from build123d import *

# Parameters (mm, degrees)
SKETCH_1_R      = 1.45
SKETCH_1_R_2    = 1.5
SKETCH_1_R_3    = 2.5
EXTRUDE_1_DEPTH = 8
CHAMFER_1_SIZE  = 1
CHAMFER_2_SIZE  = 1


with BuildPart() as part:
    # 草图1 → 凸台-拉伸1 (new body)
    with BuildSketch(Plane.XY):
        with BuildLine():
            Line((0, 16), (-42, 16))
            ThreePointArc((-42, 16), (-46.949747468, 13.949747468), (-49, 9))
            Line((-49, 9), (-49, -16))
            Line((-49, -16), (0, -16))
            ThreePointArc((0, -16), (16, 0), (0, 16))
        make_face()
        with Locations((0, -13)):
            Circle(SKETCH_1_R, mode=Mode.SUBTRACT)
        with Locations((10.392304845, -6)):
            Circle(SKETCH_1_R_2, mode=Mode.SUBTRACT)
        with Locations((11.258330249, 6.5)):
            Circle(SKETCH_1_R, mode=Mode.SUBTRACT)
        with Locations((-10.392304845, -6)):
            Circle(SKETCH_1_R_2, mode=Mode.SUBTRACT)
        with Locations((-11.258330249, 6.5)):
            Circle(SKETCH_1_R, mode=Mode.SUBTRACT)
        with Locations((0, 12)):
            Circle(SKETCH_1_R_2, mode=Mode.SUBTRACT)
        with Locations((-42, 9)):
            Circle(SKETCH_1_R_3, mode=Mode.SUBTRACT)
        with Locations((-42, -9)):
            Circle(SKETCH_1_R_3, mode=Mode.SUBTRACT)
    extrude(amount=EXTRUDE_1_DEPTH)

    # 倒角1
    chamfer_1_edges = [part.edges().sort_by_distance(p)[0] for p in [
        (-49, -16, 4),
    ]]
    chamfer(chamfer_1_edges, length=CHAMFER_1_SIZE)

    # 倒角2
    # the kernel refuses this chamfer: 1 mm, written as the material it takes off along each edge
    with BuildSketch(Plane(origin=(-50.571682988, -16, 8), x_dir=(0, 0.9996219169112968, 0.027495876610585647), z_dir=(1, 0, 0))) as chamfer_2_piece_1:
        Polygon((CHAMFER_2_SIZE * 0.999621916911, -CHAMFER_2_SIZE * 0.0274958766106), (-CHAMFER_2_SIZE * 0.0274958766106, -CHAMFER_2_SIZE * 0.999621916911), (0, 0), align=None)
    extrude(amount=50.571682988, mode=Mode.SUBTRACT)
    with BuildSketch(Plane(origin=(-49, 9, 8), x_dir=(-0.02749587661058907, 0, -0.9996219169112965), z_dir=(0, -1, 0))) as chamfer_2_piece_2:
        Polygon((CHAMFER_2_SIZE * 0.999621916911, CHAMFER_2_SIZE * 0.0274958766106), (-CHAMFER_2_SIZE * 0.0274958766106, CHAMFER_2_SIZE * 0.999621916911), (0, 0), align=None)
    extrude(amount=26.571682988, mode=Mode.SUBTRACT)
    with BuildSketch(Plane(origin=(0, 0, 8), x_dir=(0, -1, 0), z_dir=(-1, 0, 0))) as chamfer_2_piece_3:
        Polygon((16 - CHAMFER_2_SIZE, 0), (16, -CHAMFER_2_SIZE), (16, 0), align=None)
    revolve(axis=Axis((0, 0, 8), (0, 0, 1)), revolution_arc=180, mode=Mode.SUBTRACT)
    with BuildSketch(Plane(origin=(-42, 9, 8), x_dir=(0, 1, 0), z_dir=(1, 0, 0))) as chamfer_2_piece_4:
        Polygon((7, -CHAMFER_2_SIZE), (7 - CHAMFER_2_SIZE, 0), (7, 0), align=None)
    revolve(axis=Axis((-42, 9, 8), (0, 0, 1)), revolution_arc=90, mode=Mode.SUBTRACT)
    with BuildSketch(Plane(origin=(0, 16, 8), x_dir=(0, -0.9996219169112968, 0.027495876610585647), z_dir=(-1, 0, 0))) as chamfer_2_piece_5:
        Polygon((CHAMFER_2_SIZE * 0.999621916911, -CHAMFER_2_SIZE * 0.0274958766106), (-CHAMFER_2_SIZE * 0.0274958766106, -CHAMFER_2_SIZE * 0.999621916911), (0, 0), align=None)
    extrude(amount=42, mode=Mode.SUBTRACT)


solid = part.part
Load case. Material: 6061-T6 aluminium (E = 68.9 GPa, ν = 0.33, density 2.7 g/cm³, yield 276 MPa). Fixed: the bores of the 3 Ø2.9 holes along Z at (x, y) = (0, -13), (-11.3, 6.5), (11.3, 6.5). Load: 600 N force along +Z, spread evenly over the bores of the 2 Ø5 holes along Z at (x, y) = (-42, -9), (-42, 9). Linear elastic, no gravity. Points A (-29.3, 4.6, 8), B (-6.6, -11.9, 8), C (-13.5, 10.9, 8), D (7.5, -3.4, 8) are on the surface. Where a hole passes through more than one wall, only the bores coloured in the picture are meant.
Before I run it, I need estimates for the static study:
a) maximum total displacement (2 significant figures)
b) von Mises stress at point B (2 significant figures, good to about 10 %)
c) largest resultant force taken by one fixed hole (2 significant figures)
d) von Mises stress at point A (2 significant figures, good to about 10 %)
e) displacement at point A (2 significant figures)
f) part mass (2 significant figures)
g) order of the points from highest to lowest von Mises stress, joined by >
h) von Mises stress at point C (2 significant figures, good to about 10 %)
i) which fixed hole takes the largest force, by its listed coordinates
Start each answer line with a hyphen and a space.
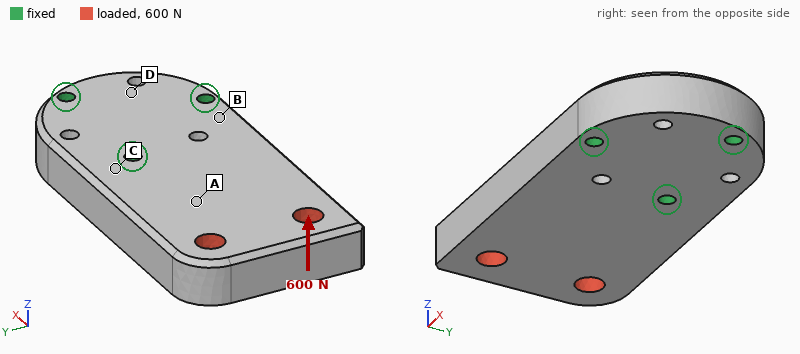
- 0.13 mm
- 33 MPa
- 910 N
- 22 MPa
- 0.043 mm
- 40 g
- C > B > A > D
- 44 MPa
- (-11.3, 6.5)
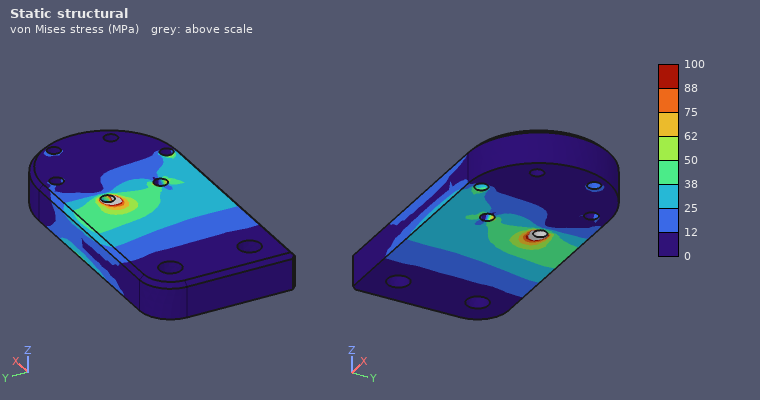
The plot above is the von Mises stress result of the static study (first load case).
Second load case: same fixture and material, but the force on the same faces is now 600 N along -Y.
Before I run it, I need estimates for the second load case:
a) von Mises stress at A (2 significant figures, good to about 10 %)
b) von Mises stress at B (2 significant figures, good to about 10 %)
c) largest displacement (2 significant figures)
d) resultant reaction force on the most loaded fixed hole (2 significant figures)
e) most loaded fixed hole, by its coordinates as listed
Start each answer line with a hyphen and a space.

- 5.8 MPa
- 12 MPa
- 15 µm
- 970 N
- (-11.3, 6.5)
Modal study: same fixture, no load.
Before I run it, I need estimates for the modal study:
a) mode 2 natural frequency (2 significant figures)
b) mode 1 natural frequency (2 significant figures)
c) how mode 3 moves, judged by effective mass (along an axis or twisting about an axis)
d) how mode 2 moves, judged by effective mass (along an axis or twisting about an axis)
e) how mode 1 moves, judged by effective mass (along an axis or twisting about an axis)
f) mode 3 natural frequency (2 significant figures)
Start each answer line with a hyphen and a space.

- 9500 Hz
- 3900 Hz
- along Y
- twisting about X
- along Z
- 10 kHz
